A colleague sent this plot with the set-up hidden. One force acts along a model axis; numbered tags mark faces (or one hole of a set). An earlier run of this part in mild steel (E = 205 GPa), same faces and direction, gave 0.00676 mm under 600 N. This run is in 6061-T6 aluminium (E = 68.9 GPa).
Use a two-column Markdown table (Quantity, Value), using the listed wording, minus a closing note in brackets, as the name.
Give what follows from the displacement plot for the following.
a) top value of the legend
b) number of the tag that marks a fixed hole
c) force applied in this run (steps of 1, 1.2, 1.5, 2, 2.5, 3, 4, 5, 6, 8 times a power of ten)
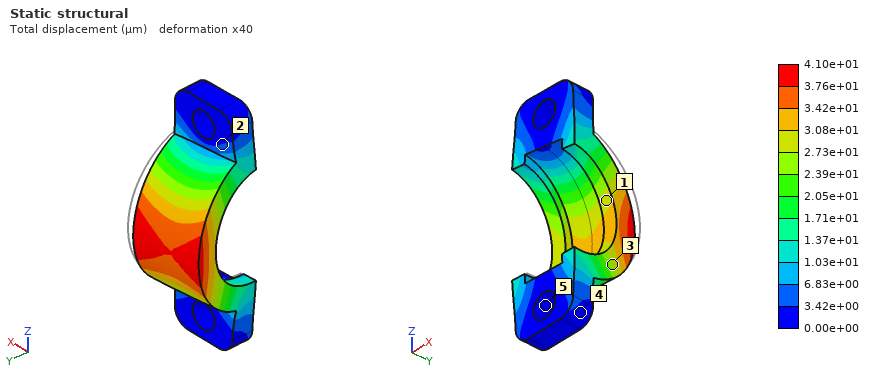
| Quantity | Value |
|---|---|
| top value of the legend | 4.10e+01 µm |
| number of the tag that marks a fixed hole | 5 |
| force applied in this run | 1.2 kN |
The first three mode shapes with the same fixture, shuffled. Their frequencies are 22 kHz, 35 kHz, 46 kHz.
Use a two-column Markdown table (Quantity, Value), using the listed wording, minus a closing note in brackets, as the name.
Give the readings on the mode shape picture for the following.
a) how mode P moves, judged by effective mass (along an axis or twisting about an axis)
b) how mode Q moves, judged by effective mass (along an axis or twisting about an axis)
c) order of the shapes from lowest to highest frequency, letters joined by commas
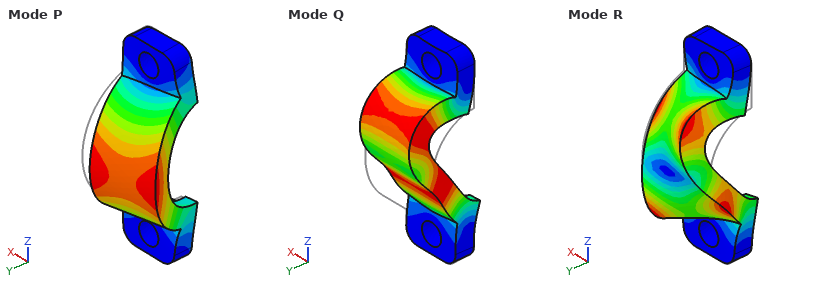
| Quantity | Value |
|---|---|
| how mode P moves, judged by effective mass | along X |
| how mode Q moves, judged by effective mass | along Z |
| order of the shapes from lowest to highest frequency, letters joined by commas | P, Q, R |
